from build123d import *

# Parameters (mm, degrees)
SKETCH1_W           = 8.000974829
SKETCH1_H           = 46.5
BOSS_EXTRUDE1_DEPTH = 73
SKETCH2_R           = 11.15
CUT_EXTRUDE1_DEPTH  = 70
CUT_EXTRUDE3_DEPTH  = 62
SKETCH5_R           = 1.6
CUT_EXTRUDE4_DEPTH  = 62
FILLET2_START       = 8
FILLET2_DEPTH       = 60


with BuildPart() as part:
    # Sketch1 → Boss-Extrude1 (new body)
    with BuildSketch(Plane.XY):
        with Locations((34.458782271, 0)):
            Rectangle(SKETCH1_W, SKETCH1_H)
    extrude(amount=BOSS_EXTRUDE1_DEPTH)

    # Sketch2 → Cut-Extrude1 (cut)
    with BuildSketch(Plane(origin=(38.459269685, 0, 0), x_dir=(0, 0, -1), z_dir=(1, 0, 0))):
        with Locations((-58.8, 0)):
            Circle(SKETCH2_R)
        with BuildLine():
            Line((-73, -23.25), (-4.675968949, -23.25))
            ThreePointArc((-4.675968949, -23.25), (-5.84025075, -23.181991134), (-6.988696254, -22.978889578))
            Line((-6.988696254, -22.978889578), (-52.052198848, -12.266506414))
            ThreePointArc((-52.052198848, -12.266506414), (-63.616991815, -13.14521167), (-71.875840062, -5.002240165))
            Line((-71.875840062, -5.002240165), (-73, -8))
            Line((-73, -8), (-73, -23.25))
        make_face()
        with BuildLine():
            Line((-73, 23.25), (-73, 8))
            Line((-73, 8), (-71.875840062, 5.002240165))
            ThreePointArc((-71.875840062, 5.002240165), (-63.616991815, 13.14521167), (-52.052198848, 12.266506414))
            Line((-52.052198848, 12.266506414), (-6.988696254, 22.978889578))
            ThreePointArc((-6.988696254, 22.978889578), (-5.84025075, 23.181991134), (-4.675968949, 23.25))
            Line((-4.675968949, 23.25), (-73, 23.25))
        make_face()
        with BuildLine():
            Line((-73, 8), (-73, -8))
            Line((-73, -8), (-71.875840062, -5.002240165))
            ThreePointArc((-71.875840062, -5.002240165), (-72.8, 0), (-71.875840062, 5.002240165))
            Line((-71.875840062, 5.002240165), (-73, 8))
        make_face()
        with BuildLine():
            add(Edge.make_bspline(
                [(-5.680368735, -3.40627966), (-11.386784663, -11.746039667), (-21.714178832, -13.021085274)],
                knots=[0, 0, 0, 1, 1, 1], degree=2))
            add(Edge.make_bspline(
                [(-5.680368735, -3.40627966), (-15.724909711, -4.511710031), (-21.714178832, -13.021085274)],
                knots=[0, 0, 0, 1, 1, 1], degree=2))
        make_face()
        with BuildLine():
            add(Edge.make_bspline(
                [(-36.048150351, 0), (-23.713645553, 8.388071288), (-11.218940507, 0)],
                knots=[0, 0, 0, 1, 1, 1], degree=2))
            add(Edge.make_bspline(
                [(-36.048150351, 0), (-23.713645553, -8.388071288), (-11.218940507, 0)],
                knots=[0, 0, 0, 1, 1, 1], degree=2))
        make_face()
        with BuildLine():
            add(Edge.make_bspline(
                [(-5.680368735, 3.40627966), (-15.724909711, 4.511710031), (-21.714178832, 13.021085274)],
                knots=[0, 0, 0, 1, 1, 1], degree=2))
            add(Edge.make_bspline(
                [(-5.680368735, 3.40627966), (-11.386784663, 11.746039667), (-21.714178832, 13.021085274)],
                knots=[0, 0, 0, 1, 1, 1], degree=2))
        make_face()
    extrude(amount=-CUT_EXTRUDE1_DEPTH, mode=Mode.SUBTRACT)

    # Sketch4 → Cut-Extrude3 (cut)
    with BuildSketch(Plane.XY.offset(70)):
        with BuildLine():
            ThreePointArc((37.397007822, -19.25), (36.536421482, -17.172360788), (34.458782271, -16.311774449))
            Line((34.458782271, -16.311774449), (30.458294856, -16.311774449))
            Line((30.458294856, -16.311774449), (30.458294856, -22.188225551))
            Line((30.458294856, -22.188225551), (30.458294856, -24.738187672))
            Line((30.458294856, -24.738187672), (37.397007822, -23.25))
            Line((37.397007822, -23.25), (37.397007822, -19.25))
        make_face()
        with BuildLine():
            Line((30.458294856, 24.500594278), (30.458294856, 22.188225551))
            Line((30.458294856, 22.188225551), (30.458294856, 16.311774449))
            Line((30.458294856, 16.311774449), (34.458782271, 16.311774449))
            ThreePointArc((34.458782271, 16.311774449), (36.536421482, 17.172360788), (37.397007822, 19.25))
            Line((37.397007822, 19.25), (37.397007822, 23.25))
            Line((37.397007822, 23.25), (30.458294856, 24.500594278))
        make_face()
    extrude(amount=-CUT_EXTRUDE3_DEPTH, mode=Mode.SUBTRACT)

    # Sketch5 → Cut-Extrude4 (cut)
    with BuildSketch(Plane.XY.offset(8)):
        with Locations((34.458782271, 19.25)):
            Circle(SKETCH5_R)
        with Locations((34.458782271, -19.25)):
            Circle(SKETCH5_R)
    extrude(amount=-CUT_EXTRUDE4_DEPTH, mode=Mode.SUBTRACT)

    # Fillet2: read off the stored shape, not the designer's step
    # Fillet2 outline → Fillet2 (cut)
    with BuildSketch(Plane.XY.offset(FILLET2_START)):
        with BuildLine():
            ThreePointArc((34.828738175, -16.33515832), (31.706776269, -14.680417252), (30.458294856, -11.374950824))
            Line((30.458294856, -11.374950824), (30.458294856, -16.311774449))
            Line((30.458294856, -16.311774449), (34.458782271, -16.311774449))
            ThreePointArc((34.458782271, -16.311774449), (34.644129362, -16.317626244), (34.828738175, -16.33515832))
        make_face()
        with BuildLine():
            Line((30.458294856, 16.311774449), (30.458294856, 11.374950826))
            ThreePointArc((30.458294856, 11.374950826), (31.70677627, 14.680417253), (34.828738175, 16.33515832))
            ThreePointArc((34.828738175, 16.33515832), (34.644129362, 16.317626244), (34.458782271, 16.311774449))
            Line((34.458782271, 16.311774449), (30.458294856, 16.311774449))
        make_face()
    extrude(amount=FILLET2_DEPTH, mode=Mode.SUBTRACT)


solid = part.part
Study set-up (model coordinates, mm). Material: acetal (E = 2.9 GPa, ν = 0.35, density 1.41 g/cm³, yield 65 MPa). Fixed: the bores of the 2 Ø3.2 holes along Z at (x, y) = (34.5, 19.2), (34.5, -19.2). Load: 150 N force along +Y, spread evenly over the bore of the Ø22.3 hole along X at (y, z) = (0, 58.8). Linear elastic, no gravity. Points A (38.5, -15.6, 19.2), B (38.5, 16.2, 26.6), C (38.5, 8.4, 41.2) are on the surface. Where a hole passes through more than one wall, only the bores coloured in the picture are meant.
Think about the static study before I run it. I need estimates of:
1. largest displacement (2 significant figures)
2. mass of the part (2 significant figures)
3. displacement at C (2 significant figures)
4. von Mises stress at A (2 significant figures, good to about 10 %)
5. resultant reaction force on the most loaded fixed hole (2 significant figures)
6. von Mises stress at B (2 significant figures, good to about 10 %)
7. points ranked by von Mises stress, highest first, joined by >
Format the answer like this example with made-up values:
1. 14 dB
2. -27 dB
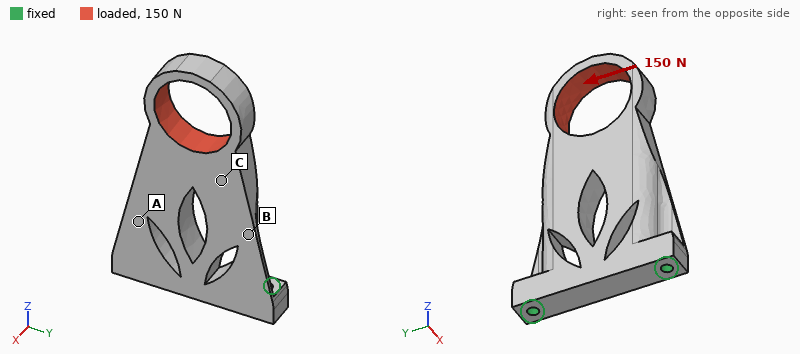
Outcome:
1. 0.81 mm
2. 18 g
3. 0.18 mm
4. 8.7 MPa
5. 240 N
6. 4.9 MPa
7. A > B > C
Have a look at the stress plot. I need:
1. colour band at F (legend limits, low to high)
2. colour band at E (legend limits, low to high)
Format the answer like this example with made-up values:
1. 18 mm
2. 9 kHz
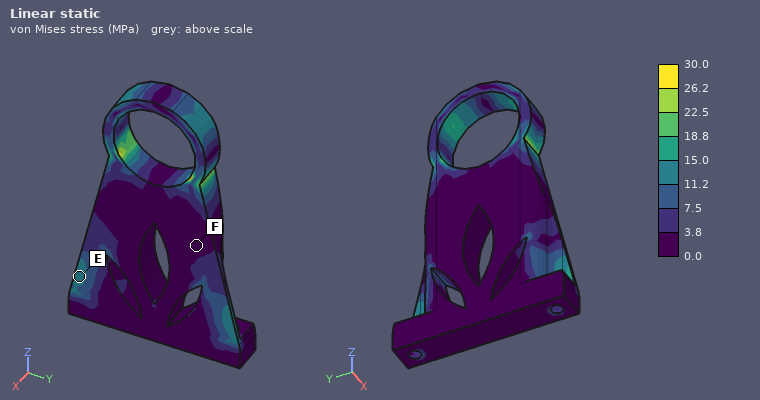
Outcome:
1. 0.0 to 3.8 MPa
2. 11.2 to 15.0 MPa
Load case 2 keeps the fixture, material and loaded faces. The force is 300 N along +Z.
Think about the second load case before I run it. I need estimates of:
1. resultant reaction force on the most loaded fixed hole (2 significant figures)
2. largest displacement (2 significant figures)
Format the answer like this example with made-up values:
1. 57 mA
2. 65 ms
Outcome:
1. 150 N
2. 0.34 mm
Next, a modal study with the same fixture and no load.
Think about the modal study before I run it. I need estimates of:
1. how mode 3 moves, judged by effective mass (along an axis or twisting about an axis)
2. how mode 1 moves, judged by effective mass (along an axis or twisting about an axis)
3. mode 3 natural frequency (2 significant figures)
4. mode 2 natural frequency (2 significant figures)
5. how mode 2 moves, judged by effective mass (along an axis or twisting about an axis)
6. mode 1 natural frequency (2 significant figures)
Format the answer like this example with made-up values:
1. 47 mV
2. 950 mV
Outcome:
1. twisting about Z
2. along X
3. 1600 Hz
4. 1400 Hz
5. along Y
6. 400 Hz
